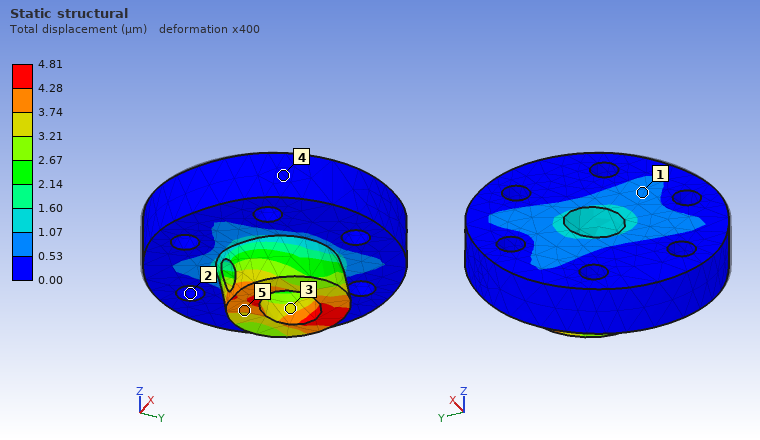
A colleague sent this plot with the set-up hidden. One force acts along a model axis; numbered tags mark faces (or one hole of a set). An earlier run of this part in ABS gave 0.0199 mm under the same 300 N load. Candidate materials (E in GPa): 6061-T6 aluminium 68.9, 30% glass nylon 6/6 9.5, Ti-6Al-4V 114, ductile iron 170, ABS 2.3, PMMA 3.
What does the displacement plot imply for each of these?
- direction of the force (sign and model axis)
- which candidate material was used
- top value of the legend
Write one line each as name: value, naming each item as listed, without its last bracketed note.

direction of the force: +Y
which candidate material was used: 30% glass nylon 6/6
top value of the legend: 4.81 µm
